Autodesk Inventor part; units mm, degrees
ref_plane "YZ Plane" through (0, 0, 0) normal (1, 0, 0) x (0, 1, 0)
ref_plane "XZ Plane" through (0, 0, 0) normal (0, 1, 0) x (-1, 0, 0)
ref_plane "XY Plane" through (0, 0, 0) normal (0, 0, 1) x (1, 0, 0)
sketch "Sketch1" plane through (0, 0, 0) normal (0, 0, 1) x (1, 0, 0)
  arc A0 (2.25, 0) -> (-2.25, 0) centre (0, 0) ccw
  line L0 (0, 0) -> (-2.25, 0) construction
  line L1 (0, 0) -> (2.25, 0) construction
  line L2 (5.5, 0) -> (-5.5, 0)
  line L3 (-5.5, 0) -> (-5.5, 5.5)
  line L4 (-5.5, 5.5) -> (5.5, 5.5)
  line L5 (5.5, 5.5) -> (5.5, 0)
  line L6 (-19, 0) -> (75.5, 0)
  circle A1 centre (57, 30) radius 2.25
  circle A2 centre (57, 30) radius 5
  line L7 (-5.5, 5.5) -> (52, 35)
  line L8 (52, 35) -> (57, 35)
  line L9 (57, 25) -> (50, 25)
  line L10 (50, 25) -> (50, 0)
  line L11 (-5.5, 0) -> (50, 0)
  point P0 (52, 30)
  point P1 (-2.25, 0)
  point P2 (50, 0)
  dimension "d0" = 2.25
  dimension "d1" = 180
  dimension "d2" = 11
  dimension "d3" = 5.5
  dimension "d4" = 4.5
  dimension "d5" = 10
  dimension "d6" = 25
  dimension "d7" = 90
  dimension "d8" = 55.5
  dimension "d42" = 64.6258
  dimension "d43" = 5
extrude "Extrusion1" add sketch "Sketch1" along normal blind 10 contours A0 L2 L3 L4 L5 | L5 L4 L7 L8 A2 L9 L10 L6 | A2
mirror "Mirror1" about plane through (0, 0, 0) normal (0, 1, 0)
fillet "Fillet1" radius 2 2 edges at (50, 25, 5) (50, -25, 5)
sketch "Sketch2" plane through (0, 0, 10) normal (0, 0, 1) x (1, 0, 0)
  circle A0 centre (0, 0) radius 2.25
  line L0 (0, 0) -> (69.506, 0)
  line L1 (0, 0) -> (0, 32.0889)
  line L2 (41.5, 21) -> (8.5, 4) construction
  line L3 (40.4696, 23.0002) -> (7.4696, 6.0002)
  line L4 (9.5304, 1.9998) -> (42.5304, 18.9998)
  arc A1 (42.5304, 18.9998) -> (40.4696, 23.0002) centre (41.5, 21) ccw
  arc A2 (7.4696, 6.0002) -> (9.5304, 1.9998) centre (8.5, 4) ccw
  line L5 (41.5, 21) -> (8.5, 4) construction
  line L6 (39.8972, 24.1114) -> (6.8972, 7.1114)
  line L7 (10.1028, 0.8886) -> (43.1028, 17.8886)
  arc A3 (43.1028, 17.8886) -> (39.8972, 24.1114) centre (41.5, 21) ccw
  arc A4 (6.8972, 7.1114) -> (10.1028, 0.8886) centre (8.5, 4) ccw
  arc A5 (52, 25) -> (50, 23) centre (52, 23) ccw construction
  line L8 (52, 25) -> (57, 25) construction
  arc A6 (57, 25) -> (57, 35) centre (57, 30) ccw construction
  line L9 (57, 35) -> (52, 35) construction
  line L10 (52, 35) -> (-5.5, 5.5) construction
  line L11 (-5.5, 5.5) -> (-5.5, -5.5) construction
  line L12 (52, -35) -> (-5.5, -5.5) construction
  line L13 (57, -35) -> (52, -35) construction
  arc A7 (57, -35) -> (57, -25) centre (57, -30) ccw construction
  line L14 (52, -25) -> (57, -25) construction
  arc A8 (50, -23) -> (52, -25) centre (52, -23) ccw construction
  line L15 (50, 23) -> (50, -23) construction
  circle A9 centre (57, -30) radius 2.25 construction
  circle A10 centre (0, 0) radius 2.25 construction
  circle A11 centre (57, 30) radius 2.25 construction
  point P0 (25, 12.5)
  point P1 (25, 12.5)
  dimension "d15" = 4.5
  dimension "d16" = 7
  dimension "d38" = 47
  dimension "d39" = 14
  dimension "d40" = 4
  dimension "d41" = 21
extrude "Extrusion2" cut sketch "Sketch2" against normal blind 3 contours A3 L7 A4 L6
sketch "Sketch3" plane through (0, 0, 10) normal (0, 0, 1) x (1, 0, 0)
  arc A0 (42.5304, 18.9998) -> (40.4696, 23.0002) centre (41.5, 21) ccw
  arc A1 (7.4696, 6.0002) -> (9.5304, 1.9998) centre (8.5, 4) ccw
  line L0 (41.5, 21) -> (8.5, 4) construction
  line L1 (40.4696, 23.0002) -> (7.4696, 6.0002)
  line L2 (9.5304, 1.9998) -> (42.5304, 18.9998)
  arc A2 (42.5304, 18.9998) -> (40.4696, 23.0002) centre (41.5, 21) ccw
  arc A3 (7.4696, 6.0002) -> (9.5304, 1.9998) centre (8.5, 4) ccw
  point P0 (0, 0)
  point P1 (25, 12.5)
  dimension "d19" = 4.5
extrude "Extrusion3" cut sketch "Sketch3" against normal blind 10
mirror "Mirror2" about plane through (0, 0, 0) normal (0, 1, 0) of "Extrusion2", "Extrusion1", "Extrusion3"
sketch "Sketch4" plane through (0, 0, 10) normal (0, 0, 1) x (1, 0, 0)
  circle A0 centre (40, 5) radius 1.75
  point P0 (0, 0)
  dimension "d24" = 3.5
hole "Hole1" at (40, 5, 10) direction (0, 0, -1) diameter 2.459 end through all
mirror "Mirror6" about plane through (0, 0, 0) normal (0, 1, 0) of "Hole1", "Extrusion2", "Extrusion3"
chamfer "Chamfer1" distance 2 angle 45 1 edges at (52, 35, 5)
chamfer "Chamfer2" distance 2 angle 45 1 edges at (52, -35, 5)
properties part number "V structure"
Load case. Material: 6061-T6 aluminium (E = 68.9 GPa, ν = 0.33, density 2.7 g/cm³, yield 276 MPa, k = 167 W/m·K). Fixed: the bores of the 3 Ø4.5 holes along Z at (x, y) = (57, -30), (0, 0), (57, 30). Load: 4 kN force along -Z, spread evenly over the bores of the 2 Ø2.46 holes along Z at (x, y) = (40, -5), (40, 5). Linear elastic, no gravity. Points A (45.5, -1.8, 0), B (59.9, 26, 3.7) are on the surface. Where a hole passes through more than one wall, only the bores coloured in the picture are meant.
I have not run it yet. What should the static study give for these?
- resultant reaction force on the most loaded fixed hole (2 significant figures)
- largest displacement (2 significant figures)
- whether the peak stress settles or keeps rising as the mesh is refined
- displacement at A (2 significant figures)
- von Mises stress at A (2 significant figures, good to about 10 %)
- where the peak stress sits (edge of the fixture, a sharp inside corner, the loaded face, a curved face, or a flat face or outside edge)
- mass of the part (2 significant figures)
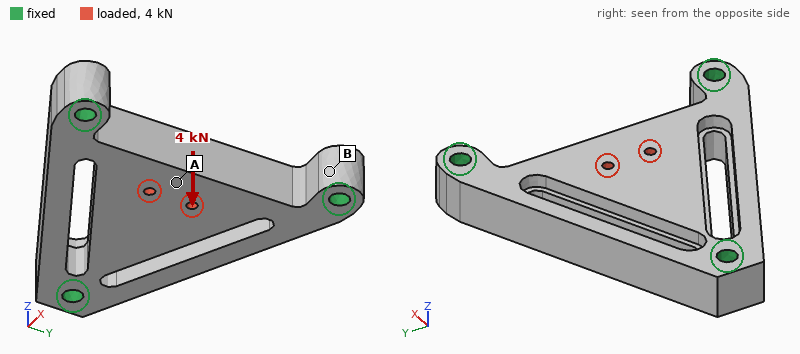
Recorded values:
1.5 kN
97 µm
keeps rising
91 µm
81 MPa
edge of the fixture
52 g
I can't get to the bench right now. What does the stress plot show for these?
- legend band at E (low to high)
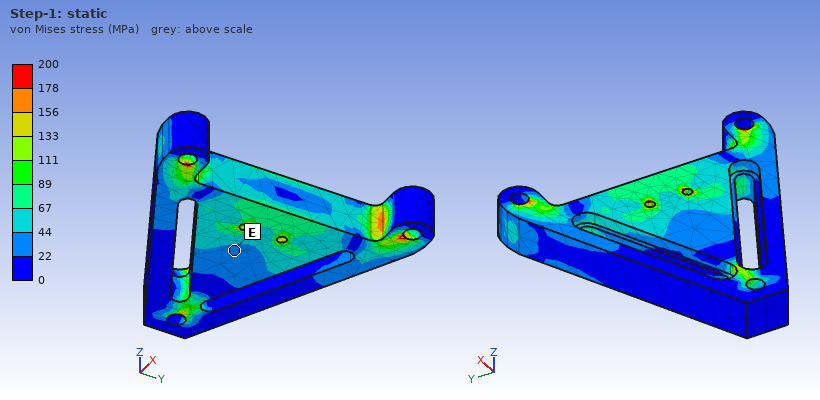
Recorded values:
22 to 44 MPa
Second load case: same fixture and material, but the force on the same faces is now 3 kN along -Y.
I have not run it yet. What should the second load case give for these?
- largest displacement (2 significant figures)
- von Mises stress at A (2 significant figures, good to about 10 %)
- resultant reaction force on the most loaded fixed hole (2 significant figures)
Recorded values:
15 µm
11 MPa
1.3 kN
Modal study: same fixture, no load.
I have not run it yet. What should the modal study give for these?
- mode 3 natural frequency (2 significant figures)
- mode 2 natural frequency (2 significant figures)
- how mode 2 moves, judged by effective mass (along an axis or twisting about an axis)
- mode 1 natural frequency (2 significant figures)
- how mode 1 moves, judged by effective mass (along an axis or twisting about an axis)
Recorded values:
11 kHz
10 kHz
along Y
7700 Hz
along Z
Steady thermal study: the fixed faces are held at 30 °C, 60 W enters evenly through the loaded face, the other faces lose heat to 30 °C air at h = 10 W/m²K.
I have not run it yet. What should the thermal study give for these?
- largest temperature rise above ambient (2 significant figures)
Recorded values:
45 K
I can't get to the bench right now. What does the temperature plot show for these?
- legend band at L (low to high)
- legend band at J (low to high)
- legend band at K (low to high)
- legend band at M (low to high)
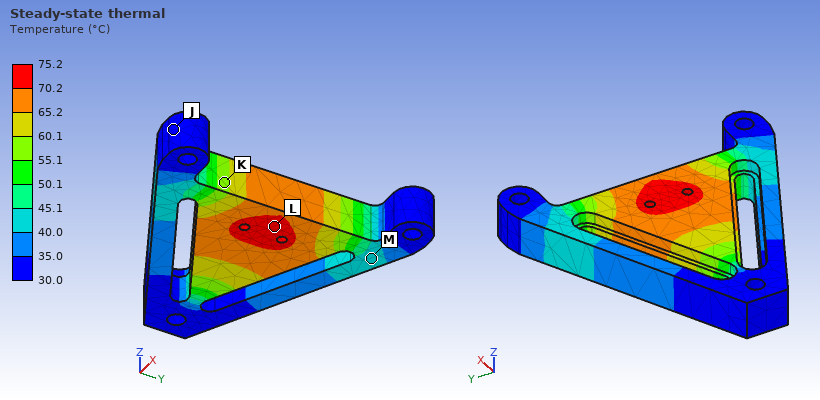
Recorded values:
70.2 to 75.2 °C
30.0 to 35.0 °C
55.1 to 60.1 °C
40.0 to 45.1 °C
